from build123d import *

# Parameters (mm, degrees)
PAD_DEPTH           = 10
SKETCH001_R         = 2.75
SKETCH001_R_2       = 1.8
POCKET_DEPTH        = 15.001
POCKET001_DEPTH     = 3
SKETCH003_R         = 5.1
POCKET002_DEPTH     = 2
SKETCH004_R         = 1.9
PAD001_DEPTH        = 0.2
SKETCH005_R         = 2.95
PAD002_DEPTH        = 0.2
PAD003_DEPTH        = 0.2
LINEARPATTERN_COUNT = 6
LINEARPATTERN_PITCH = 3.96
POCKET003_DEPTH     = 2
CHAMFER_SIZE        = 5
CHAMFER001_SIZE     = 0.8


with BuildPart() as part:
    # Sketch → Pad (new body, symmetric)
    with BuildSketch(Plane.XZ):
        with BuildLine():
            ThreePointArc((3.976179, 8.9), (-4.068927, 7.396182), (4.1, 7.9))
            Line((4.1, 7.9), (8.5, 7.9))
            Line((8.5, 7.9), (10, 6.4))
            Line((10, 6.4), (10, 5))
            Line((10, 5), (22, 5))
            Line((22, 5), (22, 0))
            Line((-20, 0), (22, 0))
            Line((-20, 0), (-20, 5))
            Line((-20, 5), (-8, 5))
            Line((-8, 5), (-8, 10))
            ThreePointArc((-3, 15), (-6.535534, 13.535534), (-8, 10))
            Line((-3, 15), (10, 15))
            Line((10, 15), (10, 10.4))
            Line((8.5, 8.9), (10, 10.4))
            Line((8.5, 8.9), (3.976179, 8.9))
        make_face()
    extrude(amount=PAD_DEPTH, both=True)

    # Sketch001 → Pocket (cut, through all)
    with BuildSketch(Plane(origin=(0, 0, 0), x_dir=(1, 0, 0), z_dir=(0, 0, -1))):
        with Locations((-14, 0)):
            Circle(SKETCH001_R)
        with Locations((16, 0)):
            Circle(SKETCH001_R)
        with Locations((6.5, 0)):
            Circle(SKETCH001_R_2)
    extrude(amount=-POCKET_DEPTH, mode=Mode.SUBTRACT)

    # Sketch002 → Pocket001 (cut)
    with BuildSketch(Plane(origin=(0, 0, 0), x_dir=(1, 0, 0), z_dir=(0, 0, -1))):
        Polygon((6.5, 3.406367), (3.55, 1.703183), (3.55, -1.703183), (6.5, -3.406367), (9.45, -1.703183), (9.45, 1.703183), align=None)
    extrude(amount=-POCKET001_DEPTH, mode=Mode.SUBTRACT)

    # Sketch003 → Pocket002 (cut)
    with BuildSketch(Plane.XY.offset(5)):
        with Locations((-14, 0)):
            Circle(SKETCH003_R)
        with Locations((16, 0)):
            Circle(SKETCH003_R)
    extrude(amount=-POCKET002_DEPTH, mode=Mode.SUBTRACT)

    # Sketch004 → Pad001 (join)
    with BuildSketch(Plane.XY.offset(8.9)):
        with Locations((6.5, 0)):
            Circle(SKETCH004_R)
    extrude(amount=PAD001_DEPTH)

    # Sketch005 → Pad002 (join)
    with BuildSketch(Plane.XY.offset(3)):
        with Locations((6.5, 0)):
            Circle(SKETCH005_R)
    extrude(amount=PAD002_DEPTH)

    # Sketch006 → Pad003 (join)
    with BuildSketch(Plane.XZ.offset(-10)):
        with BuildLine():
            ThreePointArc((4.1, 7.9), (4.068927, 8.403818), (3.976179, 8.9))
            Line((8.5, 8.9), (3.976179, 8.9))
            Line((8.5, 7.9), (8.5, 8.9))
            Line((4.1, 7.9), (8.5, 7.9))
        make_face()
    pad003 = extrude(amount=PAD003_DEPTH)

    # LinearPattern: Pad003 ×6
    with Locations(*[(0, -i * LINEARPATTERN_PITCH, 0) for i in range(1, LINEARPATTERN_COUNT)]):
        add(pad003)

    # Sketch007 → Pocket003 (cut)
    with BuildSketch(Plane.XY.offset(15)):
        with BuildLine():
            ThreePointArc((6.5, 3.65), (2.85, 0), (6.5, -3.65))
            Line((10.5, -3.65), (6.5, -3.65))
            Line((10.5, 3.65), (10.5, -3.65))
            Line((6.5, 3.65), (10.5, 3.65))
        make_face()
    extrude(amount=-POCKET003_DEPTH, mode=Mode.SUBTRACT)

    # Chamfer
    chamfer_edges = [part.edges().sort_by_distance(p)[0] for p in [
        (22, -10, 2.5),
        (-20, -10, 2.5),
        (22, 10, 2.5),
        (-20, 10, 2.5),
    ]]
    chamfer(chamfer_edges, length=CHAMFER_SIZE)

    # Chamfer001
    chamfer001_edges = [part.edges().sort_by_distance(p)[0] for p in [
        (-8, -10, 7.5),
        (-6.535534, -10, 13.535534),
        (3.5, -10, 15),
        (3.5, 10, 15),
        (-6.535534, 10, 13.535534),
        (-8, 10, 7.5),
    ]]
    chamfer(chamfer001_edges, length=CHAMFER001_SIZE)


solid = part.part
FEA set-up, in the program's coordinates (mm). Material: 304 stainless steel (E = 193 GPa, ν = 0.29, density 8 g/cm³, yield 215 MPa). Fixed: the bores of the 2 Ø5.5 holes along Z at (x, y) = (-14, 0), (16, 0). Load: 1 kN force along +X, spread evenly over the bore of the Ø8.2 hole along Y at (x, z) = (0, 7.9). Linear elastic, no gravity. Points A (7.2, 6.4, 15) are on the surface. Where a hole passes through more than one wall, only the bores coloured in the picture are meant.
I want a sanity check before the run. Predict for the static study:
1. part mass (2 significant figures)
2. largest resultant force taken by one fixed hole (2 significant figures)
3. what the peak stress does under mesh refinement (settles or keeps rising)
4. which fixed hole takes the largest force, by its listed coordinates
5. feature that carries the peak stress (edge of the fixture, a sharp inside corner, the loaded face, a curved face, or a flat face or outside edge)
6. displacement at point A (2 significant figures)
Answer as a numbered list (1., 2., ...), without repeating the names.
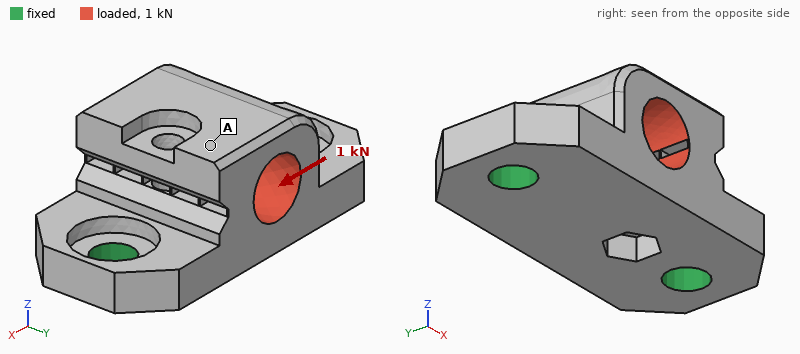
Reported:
1. 44 g
2. 590 N
3. keeps rising
4. (-14, 0)
5. a sharp inside corner
6. 2.3 µm
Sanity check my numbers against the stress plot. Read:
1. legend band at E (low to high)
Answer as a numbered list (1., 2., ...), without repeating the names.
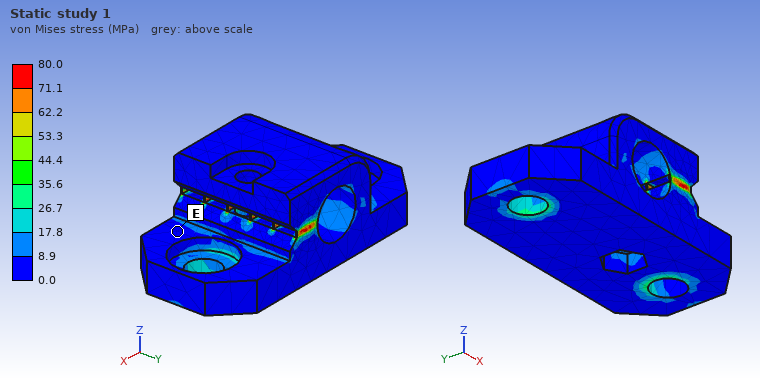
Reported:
1. 0.0 to 8.9 MPa
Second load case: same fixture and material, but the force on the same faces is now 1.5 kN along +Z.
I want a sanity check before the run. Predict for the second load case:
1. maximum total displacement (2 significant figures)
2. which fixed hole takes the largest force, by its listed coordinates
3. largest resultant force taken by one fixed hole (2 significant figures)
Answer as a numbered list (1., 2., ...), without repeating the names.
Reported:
1. 5.3 µm
2. (-14, 0)
3. 930 N
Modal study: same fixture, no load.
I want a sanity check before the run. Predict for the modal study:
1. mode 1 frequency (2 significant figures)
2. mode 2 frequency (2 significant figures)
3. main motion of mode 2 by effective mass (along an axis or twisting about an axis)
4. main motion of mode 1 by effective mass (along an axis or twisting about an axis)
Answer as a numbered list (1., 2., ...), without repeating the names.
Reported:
1. 8800 Hz
2. 17 kHz
3. along Z
4. along Y
